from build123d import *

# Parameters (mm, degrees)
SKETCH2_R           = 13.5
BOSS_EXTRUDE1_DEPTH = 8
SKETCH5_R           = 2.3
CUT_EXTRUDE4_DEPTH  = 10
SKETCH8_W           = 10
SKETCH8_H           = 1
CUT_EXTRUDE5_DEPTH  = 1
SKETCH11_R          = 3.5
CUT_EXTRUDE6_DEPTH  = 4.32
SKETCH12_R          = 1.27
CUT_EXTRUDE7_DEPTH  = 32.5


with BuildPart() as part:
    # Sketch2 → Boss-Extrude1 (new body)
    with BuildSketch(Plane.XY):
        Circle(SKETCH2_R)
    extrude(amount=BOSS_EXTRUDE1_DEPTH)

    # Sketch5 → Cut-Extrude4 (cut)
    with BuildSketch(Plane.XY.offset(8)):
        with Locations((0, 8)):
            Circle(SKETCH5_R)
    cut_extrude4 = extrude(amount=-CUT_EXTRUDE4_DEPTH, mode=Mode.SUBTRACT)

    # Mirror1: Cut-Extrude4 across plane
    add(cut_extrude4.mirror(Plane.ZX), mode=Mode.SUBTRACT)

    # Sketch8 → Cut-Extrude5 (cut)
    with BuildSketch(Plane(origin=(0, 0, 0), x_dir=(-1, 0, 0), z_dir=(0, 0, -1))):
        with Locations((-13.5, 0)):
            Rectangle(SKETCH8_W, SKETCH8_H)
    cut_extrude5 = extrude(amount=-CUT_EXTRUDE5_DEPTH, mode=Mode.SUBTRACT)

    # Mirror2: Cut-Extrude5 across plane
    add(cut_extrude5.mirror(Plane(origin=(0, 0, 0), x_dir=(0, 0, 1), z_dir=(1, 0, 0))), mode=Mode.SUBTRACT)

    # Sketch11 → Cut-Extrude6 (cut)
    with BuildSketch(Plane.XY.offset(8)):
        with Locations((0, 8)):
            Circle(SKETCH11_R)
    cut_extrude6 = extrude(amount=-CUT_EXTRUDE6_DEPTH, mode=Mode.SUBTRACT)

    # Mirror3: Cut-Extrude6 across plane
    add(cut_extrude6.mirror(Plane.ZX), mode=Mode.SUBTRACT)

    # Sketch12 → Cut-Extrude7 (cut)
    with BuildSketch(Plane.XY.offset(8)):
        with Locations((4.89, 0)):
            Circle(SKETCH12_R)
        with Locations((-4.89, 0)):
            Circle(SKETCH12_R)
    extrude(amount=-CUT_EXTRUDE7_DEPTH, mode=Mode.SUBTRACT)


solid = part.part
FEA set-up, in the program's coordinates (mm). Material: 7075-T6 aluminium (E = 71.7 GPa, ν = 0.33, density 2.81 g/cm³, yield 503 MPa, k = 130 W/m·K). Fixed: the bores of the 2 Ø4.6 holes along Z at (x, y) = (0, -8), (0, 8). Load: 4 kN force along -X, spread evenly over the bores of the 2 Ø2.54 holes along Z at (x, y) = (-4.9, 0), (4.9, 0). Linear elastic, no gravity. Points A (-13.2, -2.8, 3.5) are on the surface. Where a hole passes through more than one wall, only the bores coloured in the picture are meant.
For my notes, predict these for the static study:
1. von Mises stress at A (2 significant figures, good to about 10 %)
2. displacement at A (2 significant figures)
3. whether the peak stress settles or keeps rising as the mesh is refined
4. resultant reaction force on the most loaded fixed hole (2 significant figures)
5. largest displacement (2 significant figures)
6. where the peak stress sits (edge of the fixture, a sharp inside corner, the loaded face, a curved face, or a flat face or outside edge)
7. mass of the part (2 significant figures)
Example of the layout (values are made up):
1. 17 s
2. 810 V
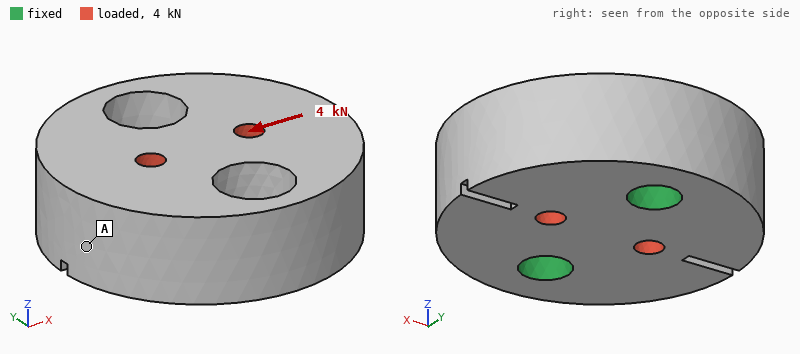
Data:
1. 16 MPa
2. 16 µm
3. keeps rising
4. 2.0 kN
5. 19 µm
6. edge of the fixture
7. 11 g
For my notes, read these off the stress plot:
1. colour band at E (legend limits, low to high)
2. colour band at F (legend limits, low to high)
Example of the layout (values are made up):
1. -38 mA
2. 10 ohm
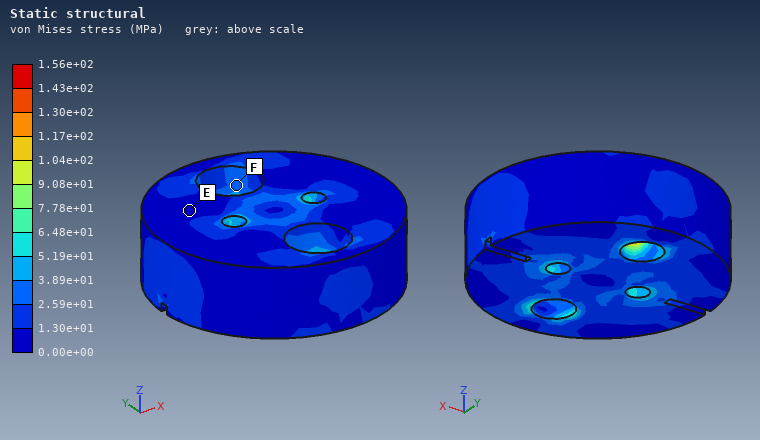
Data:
1. 0.00e+00 to 1.30e+01 MPa
2. 2.59e+01 to 3.89e+01 MPa
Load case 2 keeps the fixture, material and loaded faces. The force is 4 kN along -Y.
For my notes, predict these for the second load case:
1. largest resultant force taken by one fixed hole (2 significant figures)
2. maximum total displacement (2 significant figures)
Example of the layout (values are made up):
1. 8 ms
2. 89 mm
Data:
1. 2.1 kN
2. 5.3 µm
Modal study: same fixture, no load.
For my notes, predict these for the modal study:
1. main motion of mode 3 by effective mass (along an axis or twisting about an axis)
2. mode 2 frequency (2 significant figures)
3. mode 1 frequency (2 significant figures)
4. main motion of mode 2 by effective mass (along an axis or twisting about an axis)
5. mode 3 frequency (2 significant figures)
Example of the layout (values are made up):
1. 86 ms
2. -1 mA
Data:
1. twisting about Z
2. 31 kHz
3. 18 kHz
4. along Z
5. 44 kHz
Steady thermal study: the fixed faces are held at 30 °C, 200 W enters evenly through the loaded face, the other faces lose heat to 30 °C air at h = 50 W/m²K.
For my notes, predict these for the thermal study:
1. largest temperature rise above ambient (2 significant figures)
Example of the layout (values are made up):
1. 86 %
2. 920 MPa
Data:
1. 66 K
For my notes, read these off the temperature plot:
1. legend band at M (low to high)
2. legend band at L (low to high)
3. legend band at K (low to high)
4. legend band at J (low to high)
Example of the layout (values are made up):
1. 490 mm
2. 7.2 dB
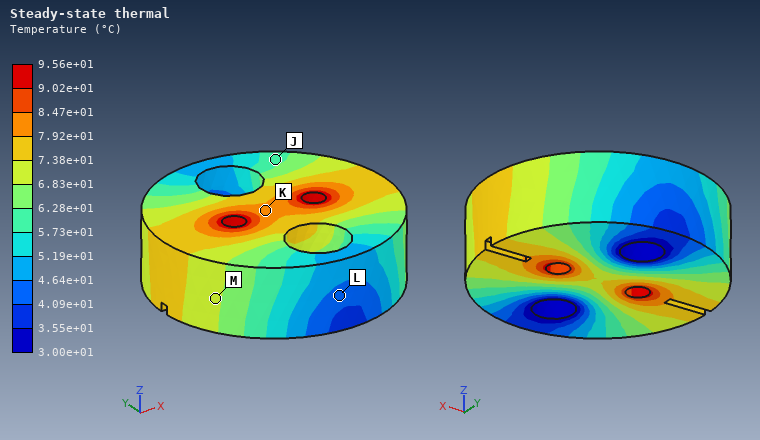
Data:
1. 6.83e+01 to 7.38e+01 °C
2. 4.09e+01 to 4.64e+01 °C
3. 7.92e+01 to 8.47e+01 °C
4. 5.73e+01 to 6.28e+01 °C
